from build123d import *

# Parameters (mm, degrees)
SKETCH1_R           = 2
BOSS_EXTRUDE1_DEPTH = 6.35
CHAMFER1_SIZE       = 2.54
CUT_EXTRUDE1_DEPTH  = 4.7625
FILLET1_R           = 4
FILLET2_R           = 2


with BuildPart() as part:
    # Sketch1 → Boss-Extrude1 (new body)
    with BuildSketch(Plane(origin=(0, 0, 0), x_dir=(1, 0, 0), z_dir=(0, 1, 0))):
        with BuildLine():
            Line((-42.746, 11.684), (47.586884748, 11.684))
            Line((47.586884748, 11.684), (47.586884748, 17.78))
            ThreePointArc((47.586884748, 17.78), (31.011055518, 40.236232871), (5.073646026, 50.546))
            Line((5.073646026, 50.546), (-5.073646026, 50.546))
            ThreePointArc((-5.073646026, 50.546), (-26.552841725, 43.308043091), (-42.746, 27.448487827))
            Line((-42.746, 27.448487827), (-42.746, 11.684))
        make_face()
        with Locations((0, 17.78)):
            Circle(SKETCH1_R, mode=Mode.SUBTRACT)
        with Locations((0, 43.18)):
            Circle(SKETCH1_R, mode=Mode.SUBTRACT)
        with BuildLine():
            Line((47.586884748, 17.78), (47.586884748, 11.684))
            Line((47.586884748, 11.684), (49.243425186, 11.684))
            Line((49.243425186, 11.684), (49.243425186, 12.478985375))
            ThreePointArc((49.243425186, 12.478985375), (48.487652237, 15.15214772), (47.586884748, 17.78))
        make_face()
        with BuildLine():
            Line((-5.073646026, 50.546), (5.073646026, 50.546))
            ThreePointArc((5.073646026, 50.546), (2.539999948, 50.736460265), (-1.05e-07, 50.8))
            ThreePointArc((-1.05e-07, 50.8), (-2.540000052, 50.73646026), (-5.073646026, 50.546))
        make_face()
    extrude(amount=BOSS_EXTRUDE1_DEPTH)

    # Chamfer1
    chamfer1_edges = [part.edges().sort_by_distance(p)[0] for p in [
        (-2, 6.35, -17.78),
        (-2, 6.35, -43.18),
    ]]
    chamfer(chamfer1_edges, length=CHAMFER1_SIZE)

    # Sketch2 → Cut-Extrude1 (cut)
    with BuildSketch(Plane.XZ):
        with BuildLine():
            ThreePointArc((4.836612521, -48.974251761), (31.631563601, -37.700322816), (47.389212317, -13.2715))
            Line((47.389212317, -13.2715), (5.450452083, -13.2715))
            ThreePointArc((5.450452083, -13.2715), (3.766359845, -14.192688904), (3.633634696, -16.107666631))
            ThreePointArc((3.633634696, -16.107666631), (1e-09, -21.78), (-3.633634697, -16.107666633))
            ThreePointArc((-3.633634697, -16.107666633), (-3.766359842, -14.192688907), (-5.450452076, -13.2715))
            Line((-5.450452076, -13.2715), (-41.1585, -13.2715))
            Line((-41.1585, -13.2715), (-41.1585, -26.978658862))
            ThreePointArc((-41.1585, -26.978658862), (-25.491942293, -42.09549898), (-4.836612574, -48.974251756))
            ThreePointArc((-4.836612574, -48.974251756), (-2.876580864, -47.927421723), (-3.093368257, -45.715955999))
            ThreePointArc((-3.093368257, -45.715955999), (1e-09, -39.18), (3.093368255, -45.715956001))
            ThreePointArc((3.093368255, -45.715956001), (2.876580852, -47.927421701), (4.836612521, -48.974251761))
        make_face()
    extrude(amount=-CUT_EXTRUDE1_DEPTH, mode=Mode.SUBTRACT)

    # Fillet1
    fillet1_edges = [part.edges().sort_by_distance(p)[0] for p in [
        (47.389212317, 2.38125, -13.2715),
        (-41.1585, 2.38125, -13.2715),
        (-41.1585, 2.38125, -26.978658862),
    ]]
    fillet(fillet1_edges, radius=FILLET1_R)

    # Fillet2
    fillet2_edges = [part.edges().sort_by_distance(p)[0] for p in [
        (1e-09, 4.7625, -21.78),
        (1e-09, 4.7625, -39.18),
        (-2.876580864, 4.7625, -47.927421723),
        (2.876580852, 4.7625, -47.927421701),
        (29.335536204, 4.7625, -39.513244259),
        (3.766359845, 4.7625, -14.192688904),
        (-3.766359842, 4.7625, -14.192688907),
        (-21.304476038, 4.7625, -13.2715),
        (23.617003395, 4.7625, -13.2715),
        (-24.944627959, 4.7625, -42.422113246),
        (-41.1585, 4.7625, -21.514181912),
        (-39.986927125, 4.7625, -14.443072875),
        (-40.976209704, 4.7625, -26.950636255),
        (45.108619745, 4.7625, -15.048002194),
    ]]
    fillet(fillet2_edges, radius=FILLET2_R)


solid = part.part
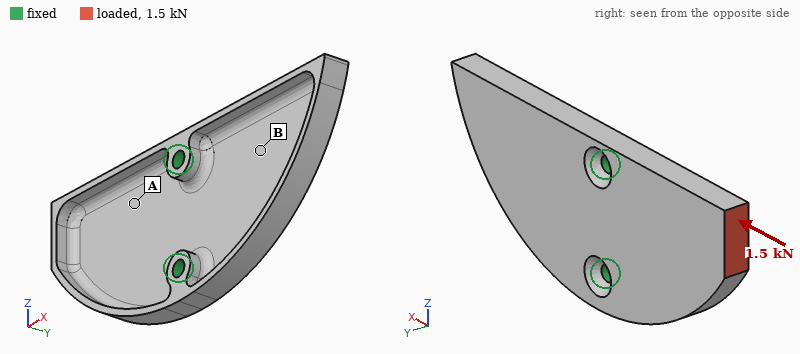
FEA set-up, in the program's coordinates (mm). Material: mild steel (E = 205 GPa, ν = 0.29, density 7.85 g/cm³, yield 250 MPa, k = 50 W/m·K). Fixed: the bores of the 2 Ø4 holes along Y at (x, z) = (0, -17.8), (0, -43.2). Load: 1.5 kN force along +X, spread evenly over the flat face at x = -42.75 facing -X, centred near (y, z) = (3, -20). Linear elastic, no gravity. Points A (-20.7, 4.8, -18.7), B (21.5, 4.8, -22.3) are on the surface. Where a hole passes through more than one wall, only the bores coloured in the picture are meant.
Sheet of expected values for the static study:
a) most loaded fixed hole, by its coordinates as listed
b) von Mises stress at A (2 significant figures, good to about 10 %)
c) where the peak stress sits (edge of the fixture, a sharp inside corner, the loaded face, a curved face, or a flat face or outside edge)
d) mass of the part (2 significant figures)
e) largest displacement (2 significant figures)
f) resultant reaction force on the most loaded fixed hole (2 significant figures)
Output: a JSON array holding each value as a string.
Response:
["(0, -17.8)", "41 MPa", "a curved face", "53 g", "0.11 mm", "1.3 kN"]
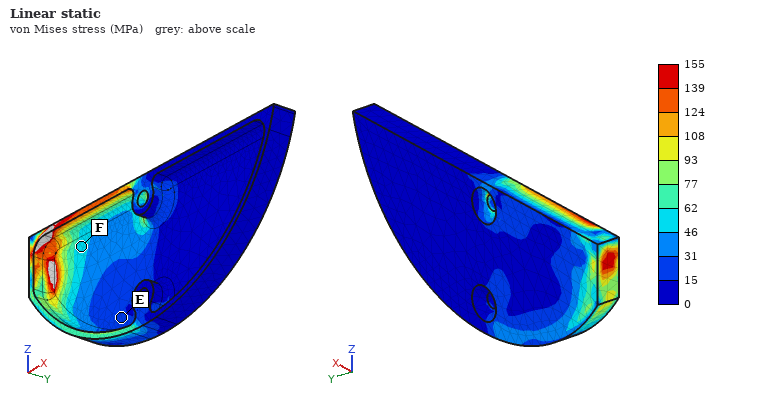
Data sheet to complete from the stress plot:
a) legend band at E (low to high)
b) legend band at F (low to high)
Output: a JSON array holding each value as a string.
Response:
["15 to 31 MPa", "46 to 62 MPa"]
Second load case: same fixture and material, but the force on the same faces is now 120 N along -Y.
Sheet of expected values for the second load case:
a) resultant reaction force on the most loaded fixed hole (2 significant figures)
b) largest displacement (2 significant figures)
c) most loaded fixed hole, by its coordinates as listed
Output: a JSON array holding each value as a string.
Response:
["89 N", "0.14 mm", "(0, -17.8)"]
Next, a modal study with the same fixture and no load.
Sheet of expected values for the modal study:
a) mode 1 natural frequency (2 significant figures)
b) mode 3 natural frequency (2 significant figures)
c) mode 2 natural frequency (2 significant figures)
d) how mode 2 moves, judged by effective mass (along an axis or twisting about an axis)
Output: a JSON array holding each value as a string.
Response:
["1600 Hz", "4300 Hz", "2100 Hz", "along Y"]
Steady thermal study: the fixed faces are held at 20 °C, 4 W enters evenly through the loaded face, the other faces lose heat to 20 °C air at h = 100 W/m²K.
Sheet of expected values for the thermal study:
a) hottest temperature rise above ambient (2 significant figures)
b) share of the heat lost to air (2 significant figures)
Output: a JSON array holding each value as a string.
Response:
["32 K", "79 %"]
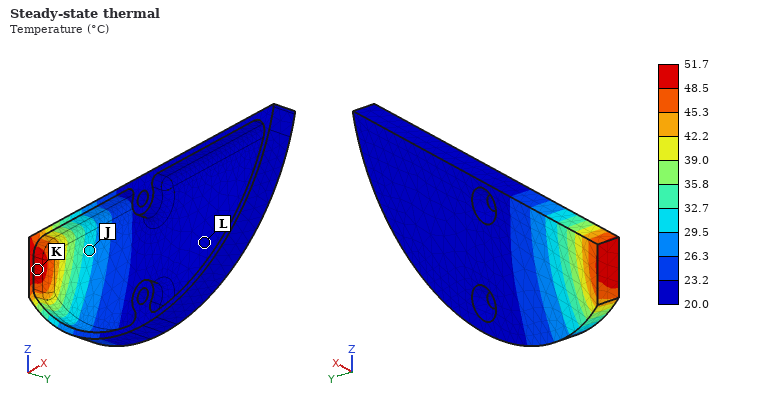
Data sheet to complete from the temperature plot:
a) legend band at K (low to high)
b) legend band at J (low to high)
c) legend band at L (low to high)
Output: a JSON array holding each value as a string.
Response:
["48.5 to 51.7 °C", "29.5 to 32.7 °C", "20.0 to 23.2 °C"]
